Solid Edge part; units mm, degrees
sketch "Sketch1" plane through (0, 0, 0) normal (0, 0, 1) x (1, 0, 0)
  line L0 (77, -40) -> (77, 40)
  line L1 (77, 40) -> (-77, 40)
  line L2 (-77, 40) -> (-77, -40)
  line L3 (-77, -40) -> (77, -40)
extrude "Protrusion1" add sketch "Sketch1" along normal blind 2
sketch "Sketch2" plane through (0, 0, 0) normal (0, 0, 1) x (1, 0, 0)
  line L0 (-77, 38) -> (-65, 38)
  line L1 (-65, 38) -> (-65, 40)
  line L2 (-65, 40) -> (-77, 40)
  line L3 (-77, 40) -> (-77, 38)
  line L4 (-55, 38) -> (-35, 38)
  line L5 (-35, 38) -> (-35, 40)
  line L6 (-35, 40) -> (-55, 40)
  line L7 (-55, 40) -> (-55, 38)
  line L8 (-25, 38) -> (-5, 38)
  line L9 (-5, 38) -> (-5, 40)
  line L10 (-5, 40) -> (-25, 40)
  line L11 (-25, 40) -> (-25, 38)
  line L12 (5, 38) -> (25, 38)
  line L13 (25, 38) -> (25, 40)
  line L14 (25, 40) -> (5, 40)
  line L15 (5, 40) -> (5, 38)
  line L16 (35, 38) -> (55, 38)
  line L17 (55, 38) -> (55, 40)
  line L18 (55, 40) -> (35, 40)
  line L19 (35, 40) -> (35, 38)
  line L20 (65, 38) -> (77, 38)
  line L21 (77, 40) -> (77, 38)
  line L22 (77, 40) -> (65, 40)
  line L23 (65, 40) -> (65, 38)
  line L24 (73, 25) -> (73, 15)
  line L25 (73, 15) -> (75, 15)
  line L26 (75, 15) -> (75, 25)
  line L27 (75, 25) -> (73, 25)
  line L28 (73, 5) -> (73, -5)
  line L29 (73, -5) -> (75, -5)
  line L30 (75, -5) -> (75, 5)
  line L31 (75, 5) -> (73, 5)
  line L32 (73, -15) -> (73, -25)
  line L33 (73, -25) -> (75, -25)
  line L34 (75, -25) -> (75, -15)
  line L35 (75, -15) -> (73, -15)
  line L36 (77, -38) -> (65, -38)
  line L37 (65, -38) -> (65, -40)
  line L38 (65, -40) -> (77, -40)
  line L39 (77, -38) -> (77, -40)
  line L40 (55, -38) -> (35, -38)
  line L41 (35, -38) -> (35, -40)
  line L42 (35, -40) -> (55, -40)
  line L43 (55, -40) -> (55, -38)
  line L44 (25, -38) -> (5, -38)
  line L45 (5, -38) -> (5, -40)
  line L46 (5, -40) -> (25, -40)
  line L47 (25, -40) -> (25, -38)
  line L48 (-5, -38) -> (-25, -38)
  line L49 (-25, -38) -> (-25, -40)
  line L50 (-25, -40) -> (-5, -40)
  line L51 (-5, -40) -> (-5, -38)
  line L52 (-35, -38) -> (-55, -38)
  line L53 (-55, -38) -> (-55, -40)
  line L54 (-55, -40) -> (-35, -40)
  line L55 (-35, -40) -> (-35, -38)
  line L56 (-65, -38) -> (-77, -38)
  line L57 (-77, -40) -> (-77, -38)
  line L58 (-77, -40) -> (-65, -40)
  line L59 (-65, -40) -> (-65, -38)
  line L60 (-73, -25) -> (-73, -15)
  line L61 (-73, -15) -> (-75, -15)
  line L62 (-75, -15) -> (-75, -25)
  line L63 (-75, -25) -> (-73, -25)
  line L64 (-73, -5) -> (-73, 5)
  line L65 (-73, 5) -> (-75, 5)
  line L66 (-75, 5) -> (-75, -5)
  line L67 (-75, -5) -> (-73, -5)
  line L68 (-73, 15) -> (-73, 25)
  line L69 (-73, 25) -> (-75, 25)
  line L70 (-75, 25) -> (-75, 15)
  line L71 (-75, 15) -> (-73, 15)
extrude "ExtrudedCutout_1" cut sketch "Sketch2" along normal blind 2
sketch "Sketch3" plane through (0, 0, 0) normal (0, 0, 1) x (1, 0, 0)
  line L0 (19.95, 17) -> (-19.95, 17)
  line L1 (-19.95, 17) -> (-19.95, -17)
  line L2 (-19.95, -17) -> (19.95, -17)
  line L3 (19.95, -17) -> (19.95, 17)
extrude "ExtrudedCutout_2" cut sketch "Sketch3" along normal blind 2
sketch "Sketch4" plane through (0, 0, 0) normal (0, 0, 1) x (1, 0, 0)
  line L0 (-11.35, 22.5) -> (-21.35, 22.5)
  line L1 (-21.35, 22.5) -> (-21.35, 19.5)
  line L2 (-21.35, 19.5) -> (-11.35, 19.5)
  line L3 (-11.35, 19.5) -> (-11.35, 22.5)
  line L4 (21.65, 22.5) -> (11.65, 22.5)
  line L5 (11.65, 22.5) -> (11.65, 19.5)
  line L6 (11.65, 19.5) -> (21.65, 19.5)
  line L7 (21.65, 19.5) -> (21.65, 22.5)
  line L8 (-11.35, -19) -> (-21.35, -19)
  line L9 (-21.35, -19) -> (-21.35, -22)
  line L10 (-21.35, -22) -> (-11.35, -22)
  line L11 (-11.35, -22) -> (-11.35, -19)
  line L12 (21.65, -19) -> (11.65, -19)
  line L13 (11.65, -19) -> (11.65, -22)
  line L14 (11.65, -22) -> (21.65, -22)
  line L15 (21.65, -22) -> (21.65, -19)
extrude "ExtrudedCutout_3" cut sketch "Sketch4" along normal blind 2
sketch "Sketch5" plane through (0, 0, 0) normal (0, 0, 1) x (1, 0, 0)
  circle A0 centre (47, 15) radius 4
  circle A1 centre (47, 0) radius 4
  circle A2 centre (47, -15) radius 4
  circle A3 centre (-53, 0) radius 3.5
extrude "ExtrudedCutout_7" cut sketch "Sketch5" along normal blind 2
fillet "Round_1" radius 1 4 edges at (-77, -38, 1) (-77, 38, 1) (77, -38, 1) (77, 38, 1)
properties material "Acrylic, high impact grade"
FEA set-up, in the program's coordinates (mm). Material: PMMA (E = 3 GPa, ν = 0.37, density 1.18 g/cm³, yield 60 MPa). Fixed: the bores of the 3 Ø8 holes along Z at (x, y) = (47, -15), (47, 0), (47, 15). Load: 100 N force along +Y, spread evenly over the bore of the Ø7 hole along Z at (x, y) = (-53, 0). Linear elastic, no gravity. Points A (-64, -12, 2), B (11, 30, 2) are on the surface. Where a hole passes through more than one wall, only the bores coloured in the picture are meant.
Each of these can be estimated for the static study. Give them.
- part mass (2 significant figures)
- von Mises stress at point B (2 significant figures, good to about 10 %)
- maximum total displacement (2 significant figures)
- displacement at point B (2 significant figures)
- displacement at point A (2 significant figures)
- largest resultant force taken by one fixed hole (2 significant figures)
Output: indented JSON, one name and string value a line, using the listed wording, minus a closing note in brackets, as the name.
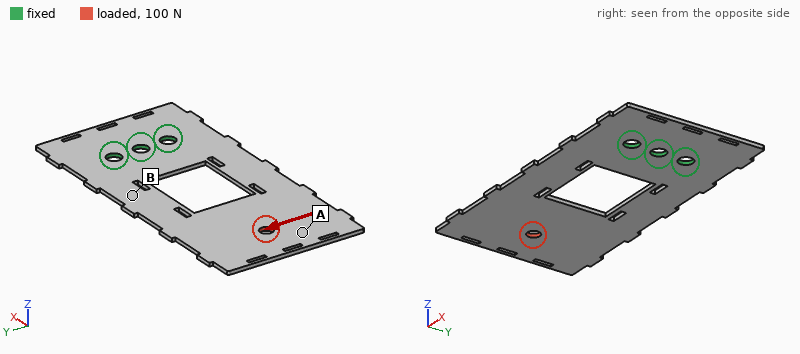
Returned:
{
  "part mass": "24 g",
  "von Mises stress at point B": "4.0 MPa",
  "maximum total displacement": "0.82 mm",
  "displacement at point B": "0.23 mm",
  "displacement at point A": "0.76 mm",
  "largest resultant force taken by one fixed hole": "260 N"
}
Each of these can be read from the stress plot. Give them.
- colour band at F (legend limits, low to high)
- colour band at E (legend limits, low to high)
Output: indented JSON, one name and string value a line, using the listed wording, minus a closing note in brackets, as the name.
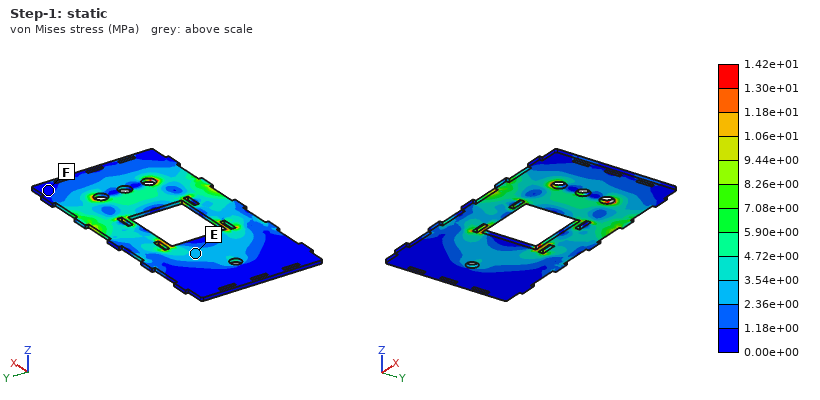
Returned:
{
  "colour band at F": "0.00e+00 to 1.18e+00 MPa",
  "colour band at E": "2.36e+00 to 3.54e+00 MPa"
}
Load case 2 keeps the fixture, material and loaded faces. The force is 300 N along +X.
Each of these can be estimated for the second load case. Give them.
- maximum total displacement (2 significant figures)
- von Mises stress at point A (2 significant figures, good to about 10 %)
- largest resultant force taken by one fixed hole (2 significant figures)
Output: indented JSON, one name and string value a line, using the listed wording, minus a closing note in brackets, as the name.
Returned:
{
  "maximum total displacement": "0.18 mm",
  "von Mises stress at point A": "2.4 MPa",
  "largest resultant force taken by one fixed hole": "140 N"
}
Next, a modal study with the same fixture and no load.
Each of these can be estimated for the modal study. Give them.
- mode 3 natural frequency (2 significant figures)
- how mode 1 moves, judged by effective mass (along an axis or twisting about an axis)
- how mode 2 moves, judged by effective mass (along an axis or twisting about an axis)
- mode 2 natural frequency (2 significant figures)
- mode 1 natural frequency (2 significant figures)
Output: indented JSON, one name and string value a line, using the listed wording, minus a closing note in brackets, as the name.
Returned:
{
  "mode 3 natural frequency": "210 Hz",
  "how mode 1 moves, judged by effective mass": "along Z",
  "how mode 2 moves, judged by effective mass": "twisting about X",
  "mode 2 natural frequency": "98 Hz",
  "mode 1 natural frequency": "29 Hz"
}
